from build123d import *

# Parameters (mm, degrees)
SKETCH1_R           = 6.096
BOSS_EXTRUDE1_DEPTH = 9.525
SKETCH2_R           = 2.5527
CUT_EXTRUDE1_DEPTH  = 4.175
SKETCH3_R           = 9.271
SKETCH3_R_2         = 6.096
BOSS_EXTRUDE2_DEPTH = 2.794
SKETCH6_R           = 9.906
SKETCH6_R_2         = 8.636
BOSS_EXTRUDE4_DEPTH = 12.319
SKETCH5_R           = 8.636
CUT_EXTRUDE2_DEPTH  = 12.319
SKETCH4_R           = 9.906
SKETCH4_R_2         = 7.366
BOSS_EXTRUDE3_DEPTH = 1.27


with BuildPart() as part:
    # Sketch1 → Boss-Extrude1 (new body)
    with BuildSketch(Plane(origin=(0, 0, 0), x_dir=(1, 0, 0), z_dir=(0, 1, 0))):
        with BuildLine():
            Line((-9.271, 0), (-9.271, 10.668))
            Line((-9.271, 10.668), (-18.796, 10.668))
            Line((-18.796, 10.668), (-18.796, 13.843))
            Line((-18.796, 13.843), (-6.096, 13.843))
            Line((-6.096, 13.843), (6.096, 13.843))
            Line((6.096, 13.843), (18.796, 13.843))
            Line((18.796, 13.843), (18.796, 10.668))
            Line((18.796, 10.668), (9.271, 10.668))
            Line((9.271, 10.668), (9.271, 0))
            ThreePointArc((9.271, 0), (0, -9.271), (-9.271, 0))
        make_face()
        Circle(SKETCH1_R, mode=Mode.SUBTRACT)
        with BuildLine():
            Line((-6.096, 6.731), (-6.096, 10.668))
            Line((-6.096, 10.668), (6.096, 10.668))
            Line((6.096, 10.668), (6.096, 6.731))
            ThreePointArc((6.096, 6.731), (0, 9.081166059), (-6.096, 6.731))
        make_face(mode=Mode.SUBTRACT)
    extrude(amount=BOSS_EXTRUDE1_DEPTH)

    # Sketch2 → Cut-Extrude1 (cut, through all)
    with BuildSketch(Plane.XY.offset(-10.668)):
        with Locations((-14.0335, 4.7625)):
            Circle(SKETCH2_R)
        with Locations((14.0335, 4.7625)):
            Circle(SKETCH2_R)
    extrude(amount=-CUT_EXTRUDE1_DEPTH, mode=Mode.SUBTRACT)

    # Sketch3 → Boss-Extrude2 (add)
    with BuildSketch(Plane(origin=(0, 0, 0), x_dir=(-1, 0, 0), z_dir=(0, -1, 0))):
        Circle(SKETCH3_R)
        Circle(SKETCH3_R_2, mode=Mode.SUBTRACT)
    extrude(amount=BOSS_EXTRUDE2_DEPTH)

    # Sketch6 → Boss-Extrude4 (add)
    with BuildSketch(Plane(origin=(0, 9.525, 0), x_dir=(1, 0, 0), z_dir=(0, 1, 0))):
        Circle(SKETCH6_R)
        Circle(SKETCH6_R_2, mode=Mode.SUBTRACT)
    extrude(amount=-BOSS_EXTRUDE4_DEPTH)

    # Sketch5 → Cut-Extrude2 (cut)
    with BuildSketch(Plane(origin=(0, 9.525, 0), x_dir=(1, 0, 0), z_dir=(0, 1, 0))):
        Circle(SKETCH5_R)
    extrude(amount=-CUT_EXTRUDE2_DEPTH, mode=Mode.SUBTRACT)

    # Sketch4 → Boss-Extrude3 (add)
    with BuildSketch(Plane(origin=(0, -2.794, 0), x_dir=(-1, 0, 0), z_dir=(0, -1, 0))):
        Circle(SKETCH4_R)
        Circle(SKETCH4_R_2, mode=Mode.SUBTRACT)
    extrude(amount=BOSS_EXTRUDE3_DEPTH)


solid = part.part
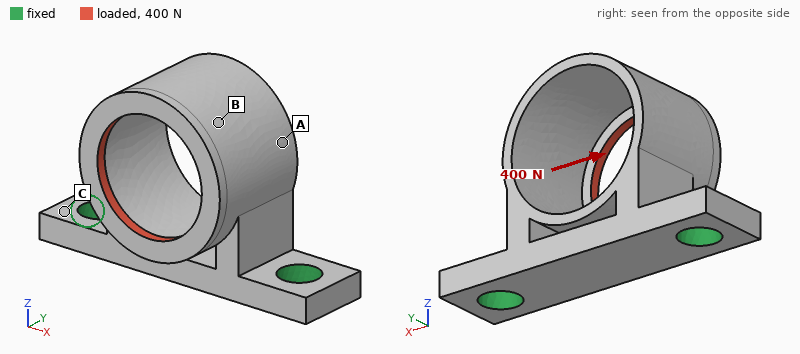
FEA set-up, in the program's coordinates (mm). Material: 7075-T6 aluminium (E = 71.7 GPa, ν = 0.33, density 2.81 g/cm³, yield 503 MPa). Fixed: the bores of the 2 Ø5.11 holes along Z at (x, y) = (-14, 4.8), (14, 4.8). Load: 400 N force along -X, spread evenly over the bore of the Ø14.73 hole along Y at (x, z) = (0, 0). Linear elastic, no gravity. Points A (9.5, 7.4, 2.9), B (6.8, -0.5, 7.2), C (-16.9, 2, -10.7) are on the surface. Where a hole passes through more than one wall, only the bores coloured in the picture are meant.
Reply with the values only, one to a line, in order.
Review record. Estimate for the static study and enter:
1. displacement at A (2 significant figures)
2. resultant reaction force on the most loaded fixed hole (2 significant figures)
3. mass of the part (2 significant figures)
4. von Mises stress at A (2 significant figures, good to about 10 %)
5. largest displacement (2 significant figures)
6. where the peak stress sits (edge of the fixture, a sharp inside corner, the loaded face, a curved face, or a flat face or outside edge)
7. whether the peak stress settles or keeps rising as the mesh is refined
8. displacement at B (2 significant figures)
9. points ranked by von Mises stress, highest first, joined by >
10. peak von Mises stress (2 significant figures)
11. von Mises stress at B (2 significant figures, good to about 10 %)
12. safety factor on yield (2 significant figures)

64 µm
320 N
6.7 g
25 MPa
95 µm
the loaded face
settles
88 µm
B > A > C
170 MPa
42 MPa
3.0
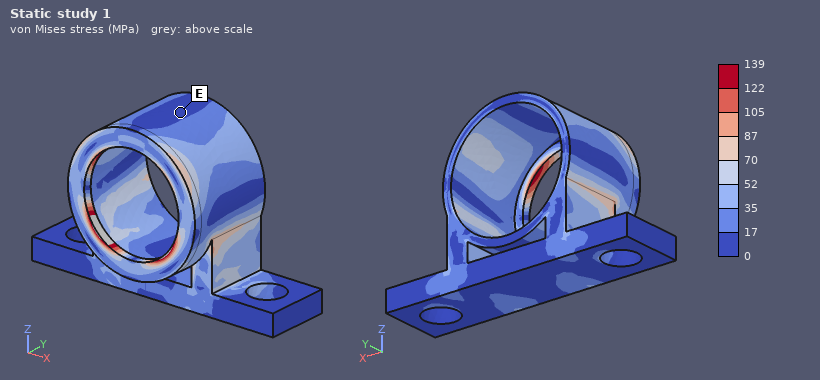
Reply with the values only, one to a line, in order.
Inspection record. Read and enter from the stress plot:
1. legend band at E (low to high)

0 to 17 MPa
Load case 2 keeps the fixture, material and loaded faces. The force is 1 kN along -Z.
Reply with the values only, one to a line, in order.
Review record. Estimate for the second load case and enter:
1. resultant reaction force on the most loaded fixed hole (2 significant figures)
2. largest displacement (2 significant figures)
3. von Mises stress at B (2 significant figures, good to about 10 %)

510 N
0.21 mm
28 MPa
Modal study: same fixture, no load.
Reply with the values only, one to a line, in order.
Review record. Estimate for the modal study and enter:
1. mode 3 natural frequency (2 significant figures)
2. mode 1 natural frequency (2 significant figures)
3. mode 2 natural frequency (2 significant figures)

14 kHz
6400 Hz
6500 Hz
